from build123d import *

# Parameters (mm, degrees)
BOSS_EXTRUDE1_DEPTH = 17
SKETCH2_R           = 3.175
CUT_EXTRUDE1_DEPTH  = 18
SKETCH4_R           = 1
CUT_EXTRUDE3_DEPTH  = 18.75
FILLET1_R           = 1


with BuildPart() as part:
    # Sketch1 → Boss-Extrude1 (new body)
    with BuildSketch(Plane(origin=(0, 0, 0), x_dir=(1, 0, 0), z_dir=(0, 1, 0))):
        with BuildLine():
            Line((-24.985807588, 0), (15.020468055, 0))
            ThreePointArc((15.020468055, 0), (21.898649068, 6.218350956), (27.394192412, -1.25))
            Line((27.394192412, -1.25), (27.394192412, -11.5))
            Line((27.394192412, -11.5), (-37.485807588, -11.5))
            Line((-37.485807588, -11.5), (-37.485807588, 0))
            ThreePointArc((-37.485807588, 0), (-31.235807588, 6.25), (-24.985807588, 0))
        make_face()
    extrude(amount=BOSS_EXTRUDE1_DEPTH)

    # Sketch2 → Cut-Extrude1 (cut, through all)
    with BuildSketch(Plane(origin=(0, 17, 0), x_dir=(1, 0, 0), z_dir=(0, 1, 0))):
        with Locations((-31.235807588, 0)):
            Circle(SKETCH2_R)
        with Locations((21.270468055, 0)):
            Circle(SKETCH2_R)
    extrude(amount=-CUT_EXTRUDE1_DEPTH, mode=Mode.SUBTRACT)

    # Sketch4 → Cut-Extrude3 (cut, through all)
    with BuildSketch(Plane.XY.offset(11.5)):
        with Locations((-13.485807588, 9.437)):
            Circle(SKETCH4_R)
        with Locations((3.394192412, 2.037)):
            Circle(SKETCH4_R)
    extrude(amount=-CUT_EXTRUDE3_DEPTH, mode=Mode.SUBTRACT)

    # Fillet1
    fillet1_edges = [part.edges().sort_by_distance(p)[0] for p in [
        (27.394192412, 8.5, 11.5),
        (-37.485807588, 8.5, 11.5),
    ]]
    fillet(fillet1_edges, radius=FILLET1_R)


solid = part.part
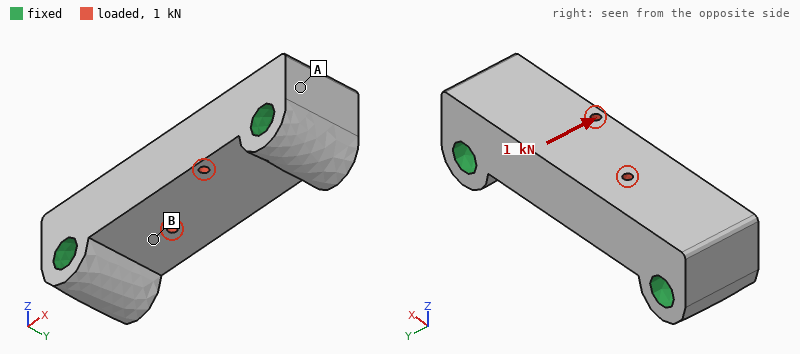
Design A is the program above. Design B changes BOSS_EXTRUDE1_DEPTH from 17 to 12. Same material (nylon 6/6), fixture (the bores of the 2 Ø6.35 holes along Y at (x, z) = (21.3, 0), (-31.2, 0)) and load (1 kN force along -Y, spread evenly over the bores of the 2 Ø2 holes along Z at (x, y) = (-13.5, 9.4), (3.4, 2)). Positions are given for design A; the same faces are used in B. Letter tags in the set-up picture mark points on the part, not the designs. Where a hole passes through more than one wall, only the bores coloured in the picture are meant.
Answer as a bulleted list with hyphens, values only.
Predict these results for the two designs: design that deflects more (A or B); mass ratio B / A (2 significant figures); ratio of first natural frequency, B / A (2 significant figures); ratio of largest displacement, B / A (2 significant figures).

- B
- 0.70
- 0.97
- 1.9
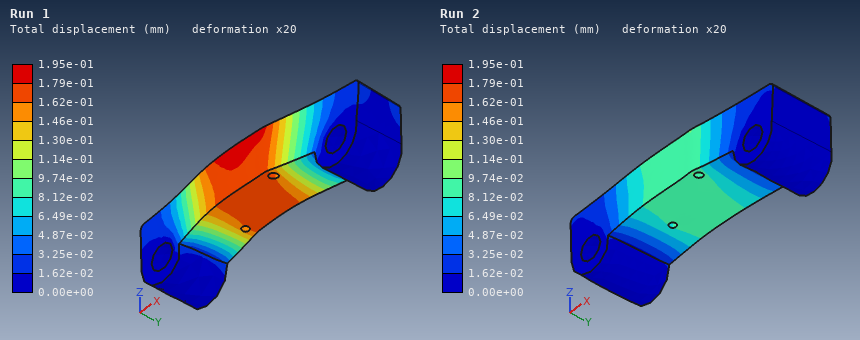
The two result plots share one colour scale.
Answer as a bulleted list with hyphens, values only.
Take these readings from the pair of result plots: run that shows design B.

- Run 1
